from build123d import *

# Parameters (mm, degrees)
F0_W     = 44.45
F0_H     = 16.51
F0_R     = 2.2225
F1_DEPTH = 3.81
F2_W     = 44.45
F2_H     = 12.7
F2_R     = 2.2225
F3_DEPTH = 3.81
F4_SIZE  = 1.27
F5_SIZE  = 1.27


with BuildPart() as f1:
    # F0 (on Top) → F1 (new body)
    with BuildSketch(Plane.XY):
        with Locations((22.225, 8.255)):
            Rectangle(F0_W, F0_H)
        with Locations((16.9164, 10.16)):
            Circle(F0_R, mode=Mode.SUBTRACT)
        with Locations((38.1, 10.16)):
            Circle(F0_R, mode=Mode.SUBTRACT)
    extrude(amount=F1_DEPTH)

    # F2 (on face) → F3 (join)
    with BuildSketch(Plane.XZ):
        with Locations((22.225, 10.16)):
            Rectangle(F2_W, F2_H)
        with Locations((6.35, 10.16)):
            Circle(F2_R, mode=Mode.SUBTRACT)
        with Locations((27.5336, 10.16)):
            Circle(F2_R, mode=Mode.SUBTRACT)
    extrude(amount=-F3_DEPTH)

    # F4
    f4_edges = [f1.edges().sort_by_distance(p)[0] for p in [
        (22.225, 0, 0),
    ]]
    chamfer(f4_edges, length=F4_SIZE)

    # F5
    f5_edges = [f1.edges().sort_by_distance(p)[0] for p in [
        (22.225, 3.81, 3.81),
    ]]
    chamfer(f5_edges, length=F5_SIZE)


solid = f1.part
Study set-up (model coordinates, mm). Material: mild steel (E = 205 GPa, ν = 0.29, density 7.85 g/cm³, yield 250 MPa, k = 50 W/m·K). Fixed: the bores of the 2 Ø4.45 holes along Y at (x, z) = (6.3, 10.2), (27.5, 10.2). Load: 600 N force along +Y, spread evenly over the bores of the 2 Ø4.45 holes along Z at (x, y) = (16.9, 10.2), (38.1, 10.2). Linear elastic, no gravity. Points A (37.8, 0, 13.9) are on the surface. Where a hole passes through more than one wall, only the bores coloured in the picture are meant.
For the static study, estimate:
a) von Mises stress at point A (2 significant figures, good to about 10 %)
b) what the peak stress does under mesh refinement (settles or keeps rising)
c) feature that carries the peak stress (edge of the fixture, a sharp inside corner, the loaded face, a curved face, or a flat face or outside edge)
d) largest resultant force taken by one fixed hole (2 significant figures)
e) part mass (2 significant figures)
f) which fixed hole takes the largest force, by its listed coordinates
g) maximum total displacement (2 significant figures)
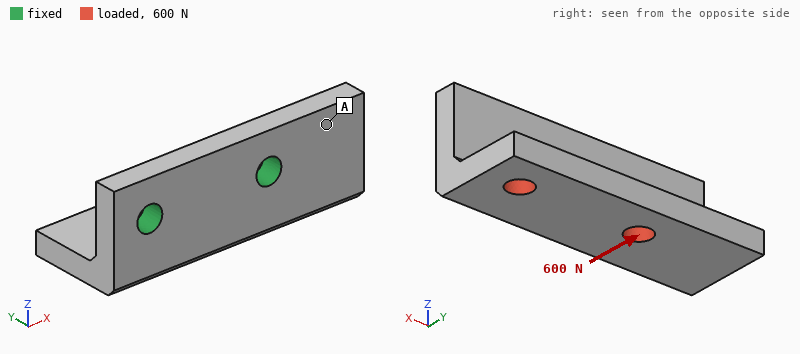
12 MPa
keeps rising
edge of the fixture
550 N
37 g
(27.5, 10.2)
15 µm
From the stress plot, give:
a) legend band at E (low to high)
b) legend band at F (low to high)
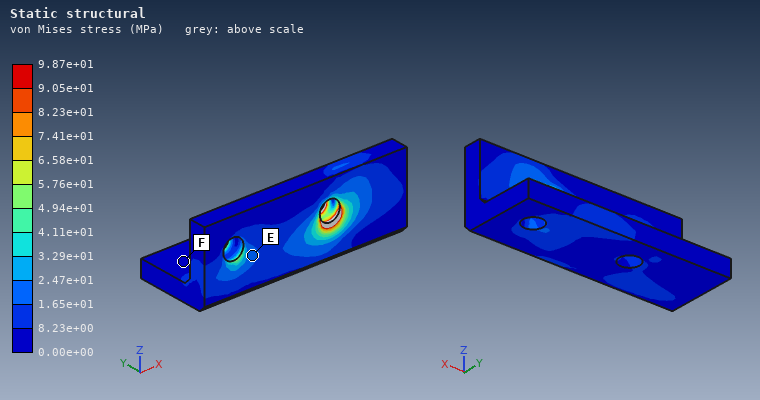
1.65e+01 to 2.47e+01 MPa
0.00e+00 to 8.23e+00 MPa
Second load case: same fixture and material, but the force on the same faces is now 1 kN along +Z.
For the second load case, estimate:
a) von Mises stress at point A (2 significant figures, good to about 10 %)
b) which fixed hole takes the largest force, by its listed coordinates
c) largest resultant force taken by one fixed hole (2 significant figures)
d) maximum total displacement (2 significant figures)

26 MPa
(27.5, 10.2)
900 N
44 µm
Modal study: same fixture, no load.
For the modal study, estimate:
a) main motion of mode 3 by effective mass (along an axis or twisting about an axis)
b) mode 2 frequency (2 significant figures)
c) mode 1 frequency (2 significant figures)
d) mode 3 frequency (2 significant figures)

along Y
11 kHz
7800 Hz
15 kHz
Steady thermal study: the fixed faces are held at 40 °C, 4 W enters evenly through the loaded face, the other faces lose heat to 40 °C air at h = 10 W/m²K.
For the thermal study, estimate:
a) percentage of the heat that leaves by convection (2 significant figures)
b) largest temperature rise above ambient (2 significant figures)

3.4 %
12 K
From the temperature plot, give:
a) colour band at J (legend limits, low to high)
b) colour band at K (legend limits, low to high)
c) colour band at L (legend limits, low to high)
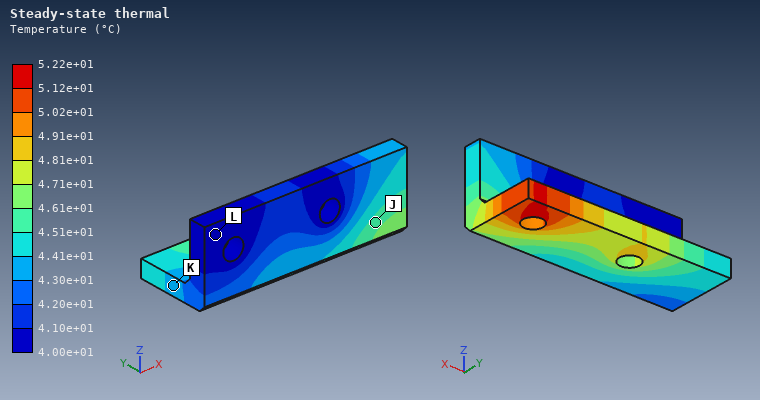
4.51e+01 to 4.61e+01 °C
4.30e+01 to 4.41e+01 °C
4.00e+01 to 4.10e+01 °C
